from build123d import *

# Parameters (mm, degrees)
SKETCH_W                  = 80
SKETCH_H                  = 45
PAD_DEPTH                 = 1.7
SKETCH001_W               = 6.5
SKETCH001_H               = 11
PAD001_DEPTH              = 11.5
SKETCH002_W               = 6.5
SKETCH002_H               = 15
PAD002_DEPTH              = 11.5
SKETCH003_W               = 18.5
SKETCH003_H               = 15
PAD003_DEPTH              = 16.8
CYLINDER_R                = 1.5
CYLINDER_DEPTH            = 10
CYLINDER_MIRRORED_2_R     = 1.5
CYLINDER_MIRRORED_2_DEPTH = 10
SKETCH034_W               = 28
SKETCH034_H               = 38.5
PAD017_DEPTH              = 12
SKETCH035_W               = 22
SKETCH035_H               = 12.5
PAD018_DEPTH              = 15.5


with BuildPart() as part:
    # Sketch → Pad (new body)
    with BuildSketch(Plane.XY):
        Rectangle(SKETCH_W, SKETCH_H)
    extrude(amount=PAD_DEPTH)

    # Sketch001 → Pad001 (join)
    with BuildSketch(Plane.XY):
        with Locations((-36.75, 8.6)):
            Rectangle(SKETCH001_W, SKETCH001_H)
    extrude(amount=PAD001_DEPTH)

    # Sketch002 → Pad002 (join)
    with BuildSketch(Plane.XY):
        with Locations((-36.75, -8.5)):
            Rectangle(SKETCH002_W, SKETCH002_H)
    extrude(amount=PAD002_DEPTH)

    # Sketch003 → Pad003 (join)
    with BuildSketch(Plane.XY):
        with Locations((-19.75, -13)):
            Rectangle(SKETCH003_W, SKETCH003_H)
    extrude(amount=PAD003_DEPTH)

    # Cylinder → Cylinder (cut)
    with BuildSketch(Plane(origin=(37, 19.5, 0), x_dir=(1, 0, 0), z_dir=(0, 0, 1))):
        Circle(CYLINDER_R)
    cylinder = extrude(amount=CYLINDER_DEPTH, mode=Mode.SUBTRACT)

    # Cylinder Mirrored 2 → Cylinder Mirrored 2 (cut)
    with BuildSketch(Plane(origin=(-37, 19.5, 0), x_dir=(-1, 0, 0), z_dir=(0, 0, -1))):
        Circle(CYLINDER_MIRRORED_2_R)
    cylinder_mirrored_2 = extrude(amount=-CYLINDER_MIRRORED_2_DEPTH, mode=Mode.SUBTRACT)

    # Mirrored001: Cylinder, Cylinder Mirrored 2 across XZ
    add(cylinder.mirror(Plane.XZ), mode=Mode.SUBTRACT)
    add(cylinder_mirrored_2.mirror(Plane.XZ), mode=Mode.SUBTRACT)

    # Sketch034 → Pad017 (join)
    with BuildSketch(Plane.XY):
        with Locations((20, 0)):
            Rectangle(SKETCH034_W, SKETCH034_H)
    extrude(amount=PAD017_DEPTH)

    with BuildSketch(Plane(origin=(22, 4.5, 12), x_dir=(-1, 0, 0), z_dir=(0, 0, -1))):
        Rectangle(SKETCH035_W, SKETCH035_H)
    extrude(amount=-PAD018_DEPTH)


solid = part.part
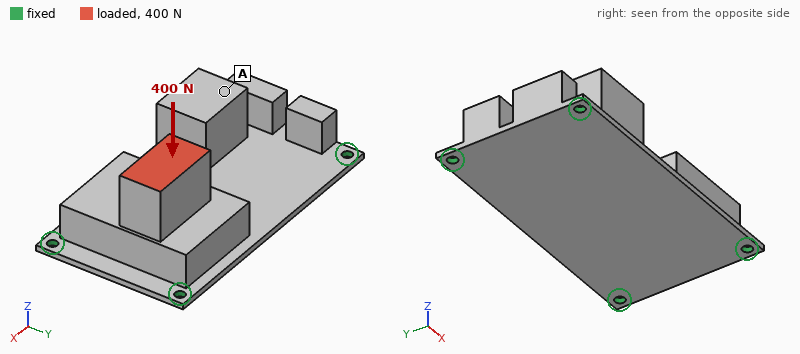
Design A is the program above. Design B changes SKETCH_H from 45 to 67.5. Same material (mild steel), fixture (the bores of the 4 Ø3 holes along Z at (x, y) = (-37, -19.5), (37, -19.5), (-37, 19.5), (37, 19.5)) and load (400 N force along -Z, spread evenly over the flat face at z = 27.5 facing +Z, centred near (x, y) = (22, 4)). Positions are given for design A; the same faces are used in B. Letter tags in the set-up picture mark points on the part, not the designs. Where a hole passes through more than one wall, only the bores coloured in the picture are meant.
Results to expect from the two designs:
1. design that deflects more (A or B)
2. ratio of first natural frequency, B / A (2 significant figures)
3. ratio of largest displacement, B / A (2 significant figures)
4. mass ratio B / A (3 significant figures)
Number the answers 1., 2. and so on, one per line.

1. A
2. 1.1
3. 0.74
4. 1.11
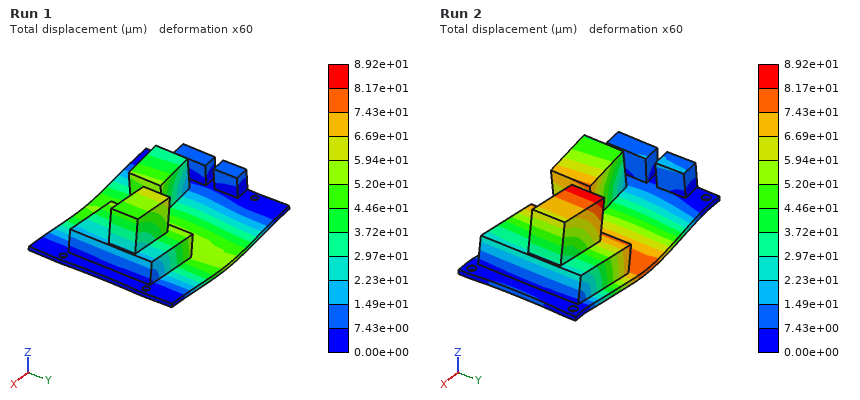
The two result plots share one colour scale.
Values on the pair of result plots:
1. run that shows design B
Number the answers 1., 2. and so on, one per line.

1. Run 1
